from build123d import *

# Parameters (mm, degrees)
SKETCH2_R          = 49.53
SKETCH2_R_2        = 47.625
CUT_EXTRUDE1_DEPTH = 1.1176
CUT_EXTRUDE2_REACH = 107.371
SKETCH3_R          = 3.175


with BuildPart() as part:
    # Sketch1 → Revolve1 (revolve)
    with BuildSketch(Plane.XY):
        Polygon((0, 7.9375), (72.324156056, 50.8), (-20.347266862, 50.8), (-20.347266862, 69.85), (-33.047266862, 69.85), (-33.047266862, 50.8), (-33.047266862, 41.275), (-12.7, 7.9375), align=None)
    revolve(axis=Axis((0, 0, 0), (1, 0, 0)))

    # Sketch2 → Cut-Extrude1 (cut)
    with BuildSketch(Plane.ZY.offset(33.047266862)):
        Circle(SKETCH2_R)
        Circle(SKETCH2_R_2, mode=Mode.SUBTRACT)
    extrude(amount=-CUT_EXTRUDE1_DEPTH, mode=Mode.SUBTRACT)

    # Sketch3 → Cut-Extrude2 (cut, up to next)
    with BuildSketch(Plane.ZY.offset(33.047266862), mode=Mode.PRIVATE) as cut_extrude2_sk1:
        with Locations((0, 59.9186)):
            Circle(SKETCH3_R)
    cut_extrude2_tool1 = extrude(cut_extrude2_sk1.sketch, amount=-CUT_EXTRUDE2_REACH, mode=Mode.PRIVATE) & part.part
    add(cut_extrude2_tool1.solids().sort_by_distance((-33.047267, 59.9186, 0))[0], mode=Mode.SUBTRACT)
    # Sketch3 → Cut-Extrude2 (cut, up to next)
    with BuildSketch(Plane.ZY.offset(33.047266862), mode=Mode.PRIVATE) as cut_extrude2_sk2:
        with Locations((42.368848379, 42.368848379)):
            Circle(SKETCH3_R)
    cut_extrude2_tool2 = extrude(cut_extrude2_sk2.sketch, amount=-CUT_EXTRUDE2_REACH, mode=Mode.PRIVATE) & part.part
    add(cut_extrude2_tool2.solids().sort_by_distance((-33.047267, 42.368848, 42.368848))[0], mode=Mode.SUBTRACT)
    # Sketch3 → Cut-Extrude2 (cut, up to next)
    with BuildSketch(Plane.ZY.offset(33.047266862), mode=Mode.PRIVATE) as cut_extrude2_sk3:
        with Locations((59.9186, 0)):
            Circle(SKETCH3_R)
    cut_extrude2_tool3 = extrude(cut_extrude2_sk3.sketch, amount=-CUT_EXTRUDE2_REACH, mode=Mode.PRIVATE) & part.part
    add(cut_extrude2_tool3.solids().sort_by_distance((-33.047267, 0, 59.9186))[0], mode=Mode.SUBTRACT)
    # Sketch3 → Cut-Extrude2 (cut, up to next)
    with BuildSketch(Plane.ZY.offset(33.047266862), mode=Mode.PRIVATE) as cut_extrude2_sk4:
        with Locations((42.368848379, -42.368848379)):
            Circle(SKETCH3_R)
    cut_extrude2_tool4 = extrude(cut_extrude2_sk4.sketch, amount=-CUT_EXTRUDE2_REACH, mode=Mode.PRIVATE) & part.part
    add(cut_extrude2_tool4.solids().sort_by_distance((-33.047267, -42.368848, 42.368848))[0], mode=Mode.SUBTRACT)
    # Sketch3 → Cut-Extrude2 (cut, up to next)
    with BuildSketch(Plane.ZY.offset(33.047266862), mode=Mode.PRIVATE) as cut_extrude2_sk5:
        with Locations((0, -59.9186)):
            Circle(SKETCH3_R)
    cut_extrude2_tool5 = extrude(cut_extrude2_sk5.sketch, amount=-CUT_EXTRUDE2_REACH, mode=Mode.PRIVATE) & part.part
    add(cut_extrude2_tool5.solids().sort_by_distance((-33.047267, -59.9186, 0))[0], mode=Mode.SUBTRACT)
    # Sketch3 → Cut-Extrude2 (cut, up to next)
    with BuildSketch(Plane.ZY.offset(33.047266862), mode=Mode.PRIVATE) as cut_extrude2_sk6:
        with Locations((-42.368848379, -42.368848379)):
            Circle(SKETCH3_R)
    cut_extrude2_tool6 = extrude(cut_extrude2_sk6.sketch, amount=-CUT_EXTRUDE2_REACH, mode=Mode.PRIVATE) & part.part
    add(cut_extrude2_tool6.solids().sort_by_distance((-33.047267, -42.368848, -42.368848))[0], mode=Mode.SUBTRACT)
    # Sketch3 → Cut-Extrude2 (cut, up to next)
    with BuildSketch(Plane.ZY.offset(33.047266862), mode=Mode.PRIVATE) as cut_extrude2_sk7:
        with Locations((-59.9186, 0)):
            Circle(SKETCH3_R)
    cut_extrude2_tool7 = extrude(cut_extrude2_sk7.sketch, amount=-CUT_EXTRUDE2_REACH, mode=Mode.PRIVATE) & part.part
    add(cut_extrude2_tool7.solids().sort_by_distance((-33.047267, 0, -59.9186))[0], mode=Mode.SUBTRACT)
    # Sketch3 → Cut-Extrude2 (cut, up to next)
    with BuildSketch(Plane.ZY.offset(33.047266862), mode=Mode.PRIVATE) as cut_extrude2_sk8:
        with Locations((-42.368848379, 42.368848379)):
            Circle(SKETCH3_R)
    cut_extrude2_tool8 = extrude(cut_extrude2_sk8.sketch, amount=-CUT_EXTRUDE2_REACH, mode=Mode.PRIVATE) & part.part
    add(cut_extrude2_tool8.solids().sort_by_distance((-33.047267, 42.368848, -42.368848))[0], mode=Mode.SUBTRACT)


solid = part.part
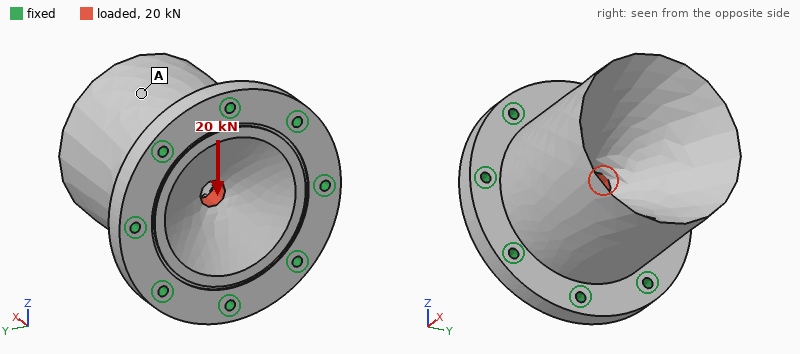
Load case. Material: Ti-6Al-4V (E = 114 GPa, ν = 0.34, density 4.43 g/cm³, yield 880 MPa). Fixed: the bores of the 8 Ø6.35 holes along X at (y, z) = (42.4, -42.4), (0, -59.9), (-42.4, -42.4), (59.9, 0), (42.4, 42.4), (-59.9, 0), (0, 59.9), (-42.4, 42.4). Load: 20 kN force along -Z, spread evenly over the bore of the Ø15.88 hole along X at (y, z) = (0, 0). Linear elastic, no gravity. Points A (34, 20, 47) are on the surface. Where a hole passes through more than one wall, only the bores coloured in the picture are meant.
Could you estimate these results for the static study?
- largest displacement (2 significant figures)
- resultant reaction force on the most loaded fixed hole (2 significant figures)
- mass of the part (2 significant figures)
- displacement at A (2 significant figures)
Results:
7.0 µm
4.0 kN
2.9 kg
5.4 µm
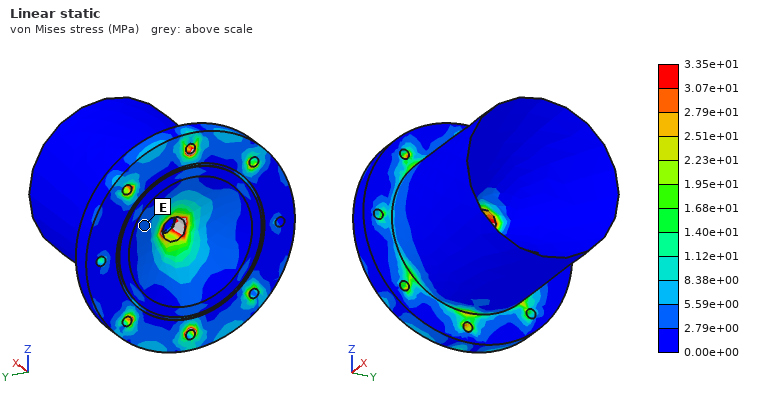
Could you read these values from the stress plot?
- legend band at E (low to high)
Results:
2.79e+00 to 5.59e+00 MPa
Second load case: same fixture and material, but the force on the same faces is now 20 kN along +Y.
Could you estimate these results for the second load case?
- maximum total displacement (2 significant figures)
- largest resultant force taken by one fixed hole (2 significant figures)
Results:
7.0 µm
4.0 kN
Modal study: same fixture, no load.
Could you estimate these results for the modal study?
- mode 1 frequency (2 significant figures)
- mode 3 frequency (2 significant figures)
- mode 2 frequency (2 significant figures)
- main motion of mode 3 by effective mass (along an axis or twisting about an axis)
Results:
4400 Hz
6400 Hz
4400 Hz
along X
